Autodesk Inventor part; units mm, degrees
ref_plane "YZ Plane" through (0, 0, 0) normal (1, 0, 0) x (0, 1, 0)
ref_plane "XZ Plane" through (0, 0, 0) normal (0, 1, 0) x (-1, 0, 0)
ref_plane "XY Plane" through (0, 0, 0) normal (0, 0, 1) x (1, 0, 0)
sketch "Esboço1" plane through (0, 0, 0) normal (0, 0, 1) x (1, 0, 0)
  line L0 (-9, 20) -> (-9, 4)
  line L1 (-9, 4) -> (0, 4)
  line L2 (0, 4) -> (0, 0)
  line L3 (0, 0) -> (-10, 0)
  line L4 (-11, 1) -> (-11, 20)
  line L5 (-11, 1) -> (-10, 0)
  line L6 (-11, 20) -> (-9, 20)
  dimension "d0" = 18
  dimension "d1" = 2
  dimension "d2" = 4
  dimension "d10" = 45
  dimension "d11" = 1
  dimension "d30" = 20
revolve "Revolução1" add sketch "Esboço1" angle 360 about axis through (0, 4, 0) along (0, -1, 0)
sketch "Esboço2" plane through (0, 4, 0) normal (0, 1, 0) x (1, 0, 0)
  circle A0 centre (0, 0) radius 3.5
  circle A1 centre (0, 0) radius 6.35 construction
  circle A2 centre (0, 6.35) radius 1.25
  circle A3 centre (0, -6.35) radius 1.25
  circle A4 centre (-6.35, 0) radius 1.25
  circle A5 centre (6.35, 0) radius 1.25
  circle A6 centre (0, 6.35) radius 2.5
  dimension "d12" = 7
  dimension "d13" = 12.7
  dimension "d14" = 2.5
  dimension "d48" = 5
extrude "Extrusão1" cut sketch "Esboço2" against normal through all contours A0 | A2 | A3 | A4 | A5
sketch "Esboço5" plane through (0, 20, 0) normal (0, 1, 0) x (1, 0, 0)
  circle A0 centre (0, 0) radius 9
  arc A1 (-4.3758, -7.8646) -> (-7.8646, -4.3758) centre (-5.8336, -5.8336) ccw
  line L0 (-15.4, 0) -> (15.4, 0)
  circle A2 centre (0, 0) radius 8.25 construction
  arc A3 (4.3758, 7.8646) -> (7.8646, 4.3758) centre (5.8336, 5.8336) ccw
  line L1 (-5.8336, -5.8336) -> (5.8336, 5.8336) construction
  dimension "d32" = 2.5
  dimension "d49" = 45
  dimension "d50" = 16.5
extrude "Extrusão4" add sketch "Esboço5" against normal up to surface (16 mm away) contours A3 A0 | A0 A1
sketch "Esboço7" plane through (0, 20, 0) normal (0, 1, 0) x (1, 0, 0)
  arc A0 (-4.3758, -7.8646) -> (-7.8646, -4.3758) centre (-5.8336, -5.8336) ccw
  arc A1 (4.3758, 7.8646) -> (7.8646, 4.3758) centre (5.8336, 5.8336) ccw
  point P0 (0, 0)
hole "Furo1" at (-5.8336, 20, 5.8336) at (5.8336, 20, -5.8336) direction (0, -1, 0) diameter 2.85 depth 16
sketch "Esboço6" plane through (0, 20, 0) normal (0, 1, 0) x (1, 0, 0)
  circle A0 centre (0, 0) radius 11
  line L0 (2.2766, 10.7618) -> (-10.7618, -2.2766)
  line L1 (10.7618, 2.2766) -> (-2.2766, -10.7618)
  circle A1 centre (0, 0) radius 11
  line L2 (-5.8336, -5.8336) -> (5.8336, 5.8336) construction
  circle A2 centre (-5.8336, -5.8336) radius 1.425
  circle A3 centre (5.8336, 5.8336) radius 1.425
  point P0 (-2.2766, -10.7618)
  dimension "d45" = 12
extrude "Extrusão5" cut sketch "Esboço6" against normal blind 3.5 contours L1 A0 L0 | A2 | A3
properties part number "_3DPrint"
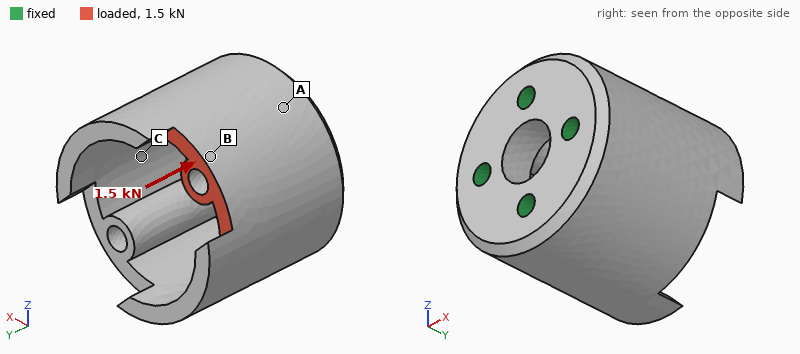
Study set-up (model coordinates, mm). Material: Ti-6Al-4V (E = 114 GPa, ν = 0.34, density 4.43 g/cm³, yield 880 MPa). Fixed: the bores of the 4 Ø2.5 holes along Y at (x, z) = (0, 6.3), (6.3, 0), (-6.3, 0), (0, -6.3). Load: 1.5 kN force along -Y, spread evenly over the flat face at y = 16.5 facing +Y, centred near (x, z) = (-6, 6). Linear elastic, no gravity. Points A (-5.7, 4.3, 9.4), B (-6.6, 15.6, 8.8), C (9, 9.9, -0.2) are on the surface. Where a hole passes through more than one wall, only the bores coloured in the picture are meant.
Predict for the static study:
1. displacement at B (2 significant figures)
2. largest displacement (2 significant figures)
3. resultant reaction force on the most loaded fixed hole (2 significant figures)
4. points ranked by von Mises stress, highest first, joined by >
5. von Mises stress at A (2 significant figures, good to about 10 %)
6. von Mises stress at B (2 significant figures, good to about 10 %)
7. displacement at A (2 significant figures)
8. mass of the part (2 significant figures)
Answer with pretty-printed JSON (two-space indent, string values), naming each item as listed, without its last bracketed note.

{
  "displacement at B": "15 µm",
  "largest displacement": "17 µm",
  "resultant reaction force on the most loaded fixed hole": "850 N",
  "points ranked by von Mises stress, highest first, joined by >": "B > A > C",
  "von Mises stress at A": "24 MPa",
  "von Mises stress at B": "45 MPa",
  "displacement at A": "6.6 µm",
  "mass of the part": "14 g"
}
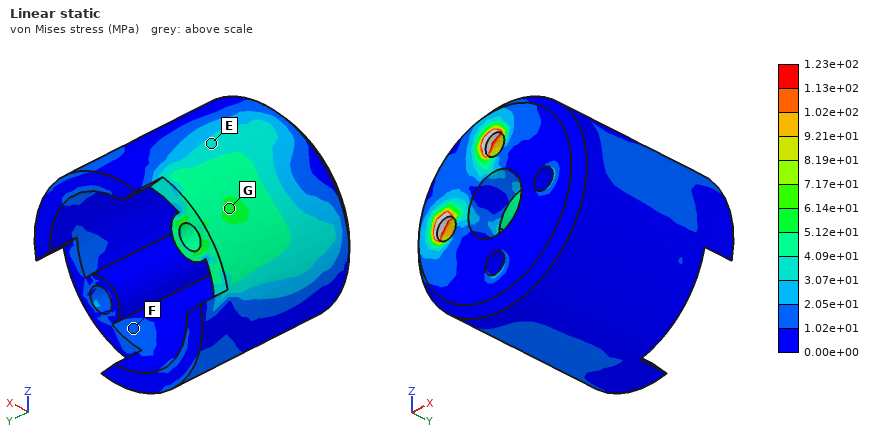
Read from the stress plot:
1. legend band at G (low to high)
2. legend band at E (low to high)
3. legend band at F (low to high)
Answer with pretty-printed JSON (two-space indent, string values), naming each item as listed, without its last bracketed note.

{
  "legend band at G": "5.12e+01 to 6.14e+01 MPa",
  "legend band at E": "3.07e+01 to 4.09e+01 MPa",
  "legend band at F": "1.02e+01 to 2.05e+01 MPa"
}
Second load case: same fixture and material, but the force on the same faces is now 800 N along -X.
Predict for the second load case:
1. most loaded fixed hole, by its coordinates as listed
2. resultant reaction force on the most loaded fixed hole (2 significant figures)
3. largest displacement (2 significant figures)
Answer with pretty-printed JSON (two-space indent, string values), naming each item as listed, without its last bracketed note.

{
  "most loaded fixed hole, by its coordinates as listed": "(-6.3, 0)",
  "resultant reaction force on the most loaded fixed hole": "780 N",
  "largest displacement": "37 µm"
}
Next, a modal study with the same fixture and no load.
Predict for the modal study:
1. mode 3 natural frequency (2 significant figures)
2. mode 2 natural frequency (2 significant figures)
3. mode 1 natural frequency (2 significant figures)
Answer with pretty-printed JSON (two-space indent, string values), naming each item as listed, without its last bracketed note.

{
  "mode 3 natural frequency": "20 kHz",
  "mode 2 natural frequency": "20 kHz",
  "mode 1 natural frequency": "17 kHz"
}
